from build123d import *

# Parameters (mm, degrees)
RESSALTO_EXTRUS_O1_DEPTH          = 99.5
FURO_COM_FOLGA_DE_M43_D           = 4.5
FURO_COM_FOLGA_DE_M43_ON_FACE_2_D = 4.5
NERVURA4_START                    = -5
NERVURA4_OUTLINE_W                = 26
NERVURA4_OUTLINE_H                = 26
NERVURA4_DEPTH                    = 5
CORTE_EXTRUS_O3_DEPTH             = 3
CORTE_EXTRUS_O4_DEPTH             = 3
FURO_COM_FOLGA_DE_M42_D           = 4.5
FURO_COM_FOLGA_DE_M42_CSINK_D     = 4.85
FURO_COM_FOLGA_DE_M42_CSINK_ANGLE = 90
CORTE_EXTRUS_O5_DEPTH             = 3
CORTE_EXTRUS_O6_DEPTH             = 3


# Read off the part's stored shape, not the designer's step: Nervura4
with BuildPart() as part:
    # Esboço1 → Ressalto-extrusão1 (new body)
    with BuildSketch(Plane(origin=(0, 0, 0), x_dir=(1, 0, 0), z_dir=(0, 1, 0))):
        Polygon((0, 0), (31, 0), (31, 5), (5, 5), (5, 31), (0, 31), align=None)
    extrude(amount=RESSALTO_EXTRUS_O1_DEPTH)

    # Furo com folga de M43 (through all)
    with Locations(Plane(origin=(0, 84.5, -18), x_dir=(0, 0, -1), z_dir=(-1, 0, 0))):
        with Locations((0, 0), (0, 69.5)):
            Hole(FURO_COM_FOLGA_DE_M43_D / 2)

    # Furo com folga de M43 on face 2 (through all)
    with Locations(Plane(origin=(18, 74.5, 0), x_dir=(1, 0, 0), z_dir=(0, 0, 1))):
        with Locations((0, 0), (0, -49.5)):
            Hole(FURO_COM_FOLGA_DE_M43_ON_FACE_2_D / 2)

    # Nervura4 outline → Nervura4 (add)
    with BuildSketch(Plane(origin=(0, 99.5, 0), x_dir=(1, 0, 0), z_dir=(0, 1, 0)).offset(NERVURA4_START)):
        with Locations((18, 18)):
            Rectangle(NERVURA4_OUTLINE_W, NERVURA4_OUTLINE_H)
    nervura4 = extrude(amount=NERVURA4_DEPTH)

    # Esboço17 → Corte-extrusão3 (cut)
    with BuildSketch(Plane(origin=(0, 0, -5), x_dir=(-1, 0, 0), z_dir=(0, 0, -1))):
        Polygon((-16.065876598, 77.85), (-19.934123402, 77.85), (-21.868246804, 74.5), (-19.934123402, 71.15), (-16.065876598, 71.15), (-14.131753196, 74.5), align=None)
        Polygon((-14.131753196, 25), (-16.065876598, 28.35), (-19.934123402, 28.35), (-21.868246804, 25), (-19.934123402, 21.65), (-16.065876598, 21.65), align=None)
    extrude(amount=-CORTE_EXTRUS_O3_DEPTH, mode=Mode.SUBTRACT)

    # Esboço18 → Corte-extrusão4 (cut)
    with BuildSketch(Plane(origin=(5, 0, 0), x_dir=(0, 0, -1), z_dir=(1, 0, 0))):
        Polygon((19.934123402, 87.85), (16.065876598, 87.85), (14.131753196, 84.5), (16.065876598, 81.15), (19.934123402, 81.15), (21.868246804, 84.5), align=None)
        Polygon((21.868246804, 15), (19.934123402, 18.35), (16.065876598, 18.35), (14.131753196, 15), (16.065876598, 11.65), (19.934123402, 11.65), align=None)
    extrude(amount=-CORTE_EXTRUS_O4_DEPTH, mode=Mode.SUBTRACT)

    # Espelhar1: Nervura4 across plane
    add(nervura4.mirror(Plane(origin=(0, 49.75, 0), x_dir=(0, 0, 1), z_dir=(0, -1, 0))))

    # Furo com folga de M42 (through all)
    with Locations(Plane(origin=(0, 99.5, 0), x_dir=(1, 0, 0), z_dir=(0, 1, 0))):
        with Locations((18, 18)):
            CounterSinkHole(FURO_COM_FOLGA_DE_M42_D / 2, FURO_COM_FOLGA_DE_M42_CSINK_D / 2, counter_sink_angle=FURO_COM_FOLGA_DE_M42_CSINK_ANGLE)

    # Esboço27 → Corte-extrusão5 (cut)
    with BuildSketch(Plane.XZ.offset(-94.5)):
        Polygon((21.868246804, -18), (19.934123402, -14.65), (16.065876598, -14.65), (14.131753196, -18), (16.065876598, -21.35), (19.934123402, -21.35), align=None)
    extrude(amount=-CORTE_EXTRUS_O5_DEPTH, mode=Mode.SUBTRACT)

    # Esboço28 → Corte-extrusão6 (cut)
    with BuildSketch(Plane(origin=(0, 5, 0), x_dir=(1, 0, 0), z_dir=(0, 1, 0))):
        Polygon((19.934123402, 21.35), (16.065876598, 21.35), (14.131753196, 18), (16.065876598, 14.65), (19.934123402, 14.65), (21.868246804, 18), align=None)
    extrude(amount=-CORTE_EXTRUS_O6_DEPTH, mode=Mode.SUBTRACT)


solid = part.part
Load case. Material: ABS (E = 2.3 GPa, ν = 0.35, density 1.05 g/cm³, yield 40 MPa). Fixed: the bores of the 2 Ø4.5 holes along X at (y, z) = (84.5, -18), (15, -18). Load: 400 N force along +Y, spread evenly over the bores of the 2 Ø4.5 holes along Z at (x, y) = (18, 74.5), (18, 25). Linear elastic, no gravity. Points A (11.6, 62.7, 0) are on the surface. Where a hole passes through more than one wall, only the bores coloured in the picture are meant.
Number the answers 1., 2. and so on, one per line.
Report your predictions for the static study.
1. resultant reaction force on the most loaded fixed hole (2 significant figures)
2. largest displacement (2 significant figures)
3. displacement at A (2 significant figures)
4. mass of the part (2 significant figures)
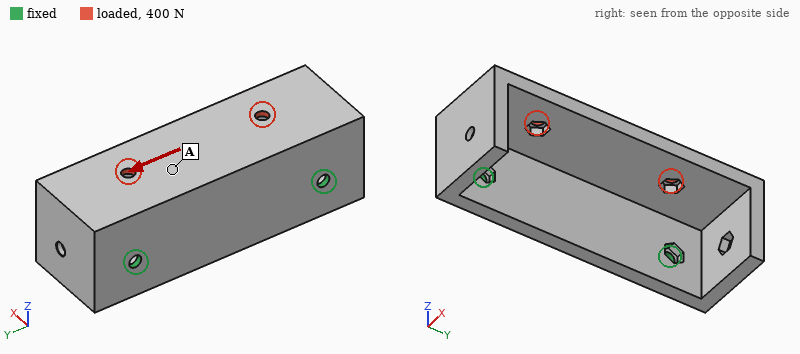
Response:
1. 240 N
2. 0.46 mm
3. 0.12 mm
4. 36 g
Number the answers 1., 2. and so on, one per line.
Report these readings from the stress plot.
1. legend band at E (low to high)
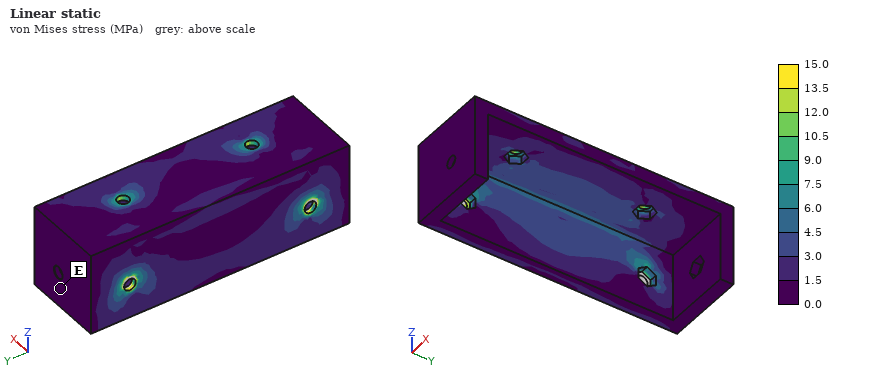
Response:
1. 0.0 to 1.5 MPa
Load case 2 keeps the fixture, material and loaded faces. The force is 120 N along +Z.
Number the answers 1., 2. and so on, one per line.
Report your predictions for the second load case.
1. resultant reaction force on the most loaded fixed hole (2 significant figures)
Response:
1. 62 N
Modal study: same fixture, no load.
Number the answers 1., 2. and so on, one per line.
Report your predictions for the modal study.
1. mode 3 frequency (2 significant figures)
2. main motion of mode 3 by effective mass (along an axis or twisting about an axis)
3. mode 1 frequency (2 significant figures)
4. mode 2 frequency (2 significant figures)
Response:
1. 1500 Hz
2. along X
3. 410 Hz
4. 710 Hz
